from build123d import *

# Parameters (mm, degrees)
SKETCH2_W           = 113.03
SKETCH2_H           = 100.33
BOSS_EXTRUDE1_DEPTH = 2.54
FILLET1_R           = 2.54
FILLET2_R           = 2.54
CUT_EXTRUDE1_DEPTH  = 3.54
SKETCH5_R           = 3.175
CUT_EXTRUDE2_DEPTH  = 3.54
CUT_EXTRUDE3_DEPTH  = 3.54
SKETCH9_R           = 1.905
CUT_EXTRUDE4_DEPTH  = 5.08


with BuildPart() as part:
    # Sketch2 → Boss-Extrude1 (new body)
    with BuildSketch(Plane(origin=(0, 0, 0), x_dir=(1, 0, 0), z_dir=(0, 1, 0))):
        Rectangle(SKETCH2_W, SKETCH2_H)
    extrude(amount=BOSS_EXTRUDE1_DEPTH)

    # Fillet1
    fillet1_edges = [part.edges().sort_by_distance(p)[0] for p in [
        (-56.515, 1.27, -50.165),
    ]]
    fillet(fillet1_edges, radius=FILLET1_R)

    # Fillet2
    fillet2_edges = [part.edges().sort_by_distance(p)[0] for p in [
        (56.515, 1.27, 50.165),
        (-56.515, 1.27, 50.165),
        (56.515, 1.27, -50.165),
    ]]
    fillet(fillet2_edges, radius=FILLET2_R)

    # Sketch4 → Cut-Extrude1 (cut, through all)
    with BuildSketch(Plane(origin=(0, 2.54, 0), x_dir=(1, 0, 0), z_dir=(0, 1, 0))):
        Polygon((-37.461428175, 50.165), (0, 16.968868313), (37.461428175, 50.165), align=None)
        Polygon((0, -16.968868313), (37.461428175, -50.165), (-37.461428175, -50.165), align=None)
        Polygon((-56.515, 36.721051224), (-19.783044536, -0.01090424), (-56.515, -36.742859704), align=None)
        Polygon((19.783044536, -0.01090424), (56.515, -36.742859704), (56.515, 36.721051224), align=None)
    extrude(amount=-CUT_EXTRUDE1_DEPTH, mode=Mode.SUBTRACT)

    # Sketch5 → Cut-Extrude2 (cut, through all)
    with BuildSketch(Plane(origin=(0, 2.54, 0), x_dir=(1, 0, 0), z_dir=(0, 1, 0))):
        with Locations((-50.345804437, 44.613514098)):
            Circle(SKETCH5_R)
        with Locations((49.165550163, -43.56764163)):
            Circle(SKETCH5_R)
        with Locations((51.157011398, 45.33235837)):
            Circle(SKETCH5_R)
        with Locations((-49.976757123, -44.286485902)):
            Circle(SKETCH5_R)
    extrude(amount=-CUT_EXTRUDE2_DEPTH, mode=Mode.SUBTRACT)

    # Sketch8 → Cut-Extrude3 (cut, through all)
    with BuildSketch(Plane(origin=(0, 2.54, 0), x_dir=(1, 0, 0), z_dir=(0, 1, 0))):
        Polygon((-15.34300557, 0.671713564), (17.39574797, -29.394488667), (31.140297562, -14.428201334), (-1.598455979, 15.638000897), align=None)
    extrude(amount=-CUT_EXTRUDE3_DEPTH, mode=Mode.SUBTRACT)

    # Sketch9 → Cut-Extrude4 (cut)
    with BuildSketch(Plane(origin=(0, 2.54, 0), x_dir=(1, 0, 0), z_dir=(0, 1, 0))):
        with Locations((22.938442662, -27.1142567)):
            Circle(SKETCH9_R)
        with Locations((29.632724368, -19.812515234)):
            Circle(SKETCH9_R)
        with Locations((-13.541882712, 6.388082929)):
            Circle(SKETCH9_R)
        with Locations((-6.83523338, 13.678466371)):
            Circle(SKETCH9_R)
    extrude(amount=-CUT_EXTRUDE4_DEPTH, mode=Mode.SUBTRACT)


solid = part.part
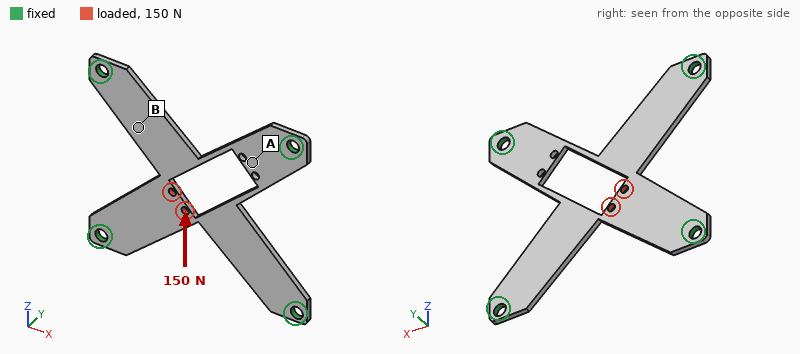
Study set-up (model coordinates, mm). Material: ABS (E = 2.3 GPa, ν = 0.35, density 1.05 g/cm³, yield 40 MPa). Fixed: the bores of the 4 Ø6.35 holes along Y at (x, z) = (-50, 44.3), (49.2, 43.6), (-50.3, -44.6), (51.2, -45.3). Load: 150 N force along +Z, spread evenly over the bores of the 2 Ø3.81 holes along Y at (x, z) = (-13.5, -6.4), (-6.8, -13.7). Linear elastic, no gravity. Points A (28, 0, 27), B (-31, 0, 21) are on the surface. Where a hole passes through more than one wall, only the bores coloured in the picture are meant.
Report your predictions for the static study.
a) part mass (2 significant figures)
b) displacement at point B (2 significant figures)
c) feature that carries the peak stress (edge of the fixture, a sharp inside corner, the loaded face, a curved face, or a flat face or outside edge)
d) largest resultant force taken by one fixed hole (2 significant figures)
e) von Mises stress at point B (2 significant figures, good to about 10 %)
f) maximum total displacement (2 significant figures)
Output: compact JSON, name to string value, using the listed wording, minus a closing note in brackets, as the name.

{"part mass": "14 g", "displacement at point B": "0.036 mm", "feature that carries the peak stress": "the loaded face", "largest resultant force taken by one fixed hole": "82 N", "von Mises stress at point B": "2.0 MPa", "maximum total displacement": "0.11 mm"}
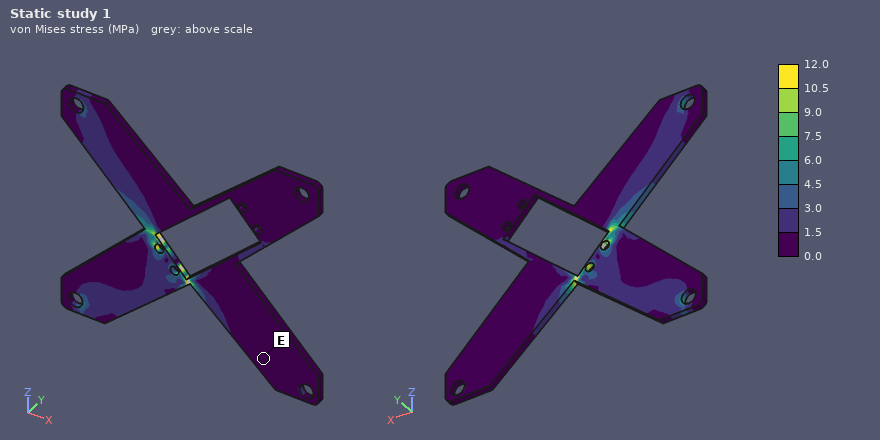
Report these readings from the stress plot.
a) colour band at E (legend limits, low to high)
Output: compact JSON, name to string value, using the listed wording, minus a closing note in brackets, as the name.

{"colour band at E": "0.0 to 1.5 MPa"}
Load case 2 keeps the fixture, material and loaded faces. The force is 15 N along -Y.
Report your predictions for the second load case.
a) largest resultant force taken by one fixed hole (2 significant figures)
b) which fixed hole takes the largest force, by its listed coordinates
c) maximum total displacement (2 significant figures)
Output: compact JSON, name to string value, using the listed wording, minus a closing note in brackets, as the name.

{"largest resultant force taken by one fixed hole": "6.4 N", "which fixed hole takes the largest force, by its listed coordinates": "(-50.3, -44.6)", "maximum total displacement": "1.8 mm"}
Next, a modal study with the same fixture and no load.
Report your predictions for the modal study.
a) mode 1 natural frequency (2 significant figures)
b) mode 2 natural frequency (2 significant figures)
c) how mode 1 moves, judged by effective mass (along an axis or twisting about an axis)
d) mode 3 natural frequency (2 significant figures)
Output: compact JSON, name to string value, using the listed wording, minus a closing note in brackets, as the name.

{"mode 1 natural frequency": "270 Hz", "mode 2 natural frequency": "530 Hz", "how mode 1 moves, judged by effective mass": "along Y", "mode 3 natural frequency": "660 Hz"}
